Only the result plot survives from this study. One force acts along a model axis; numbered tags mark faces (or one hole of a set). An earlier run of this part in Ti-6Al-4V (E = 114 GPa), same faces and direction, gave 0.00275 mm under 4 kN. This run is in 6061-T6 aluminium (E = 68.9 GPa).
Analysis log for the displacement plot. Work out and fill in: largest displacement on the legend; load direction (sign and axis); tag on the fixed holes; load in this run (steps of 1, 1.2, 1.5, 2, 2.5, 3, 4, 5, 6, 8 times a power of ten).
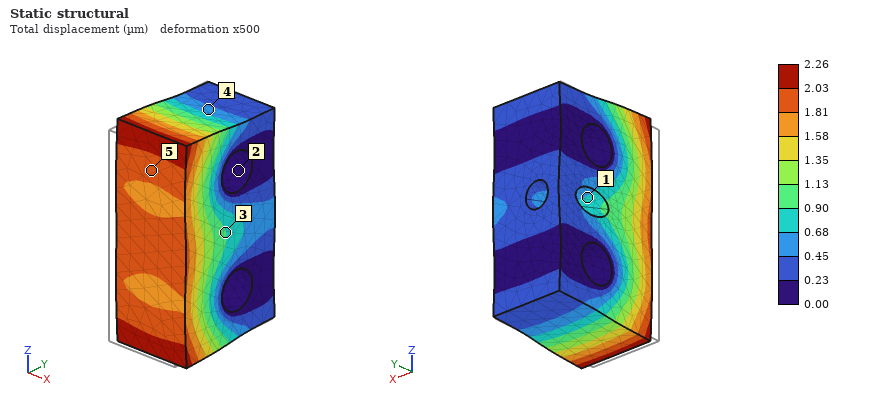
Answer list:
2.26 µm
+Y
2
2 kN
